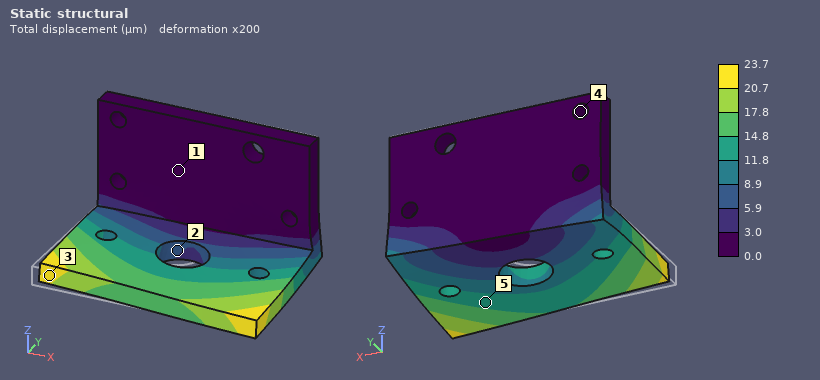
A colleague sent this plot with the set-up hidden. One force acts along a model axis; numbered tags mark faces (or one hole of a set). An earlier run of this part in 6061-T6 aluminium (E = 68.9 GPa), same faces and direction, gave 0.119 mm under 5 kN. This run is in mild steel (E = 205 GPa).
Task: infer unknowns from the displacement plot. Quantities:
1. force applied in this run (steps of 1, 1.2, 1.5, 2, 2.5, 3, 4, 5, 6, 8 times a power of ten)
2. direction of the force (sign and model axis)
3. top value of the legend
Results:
3 kN
+X
23.7 µm
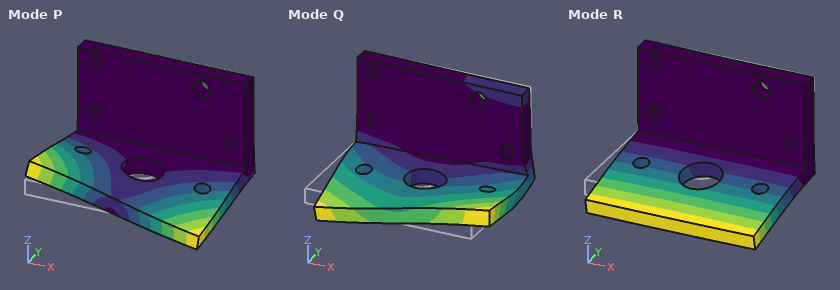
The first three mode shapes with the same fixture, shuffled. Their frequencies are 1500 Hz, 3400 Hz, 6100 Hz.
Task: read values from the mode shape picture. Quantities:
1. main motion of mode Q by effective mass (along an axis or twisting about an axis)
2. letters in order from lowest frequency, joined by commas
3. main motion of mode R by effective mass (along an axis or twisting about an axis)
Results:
along X
R, P, Q
along Z
